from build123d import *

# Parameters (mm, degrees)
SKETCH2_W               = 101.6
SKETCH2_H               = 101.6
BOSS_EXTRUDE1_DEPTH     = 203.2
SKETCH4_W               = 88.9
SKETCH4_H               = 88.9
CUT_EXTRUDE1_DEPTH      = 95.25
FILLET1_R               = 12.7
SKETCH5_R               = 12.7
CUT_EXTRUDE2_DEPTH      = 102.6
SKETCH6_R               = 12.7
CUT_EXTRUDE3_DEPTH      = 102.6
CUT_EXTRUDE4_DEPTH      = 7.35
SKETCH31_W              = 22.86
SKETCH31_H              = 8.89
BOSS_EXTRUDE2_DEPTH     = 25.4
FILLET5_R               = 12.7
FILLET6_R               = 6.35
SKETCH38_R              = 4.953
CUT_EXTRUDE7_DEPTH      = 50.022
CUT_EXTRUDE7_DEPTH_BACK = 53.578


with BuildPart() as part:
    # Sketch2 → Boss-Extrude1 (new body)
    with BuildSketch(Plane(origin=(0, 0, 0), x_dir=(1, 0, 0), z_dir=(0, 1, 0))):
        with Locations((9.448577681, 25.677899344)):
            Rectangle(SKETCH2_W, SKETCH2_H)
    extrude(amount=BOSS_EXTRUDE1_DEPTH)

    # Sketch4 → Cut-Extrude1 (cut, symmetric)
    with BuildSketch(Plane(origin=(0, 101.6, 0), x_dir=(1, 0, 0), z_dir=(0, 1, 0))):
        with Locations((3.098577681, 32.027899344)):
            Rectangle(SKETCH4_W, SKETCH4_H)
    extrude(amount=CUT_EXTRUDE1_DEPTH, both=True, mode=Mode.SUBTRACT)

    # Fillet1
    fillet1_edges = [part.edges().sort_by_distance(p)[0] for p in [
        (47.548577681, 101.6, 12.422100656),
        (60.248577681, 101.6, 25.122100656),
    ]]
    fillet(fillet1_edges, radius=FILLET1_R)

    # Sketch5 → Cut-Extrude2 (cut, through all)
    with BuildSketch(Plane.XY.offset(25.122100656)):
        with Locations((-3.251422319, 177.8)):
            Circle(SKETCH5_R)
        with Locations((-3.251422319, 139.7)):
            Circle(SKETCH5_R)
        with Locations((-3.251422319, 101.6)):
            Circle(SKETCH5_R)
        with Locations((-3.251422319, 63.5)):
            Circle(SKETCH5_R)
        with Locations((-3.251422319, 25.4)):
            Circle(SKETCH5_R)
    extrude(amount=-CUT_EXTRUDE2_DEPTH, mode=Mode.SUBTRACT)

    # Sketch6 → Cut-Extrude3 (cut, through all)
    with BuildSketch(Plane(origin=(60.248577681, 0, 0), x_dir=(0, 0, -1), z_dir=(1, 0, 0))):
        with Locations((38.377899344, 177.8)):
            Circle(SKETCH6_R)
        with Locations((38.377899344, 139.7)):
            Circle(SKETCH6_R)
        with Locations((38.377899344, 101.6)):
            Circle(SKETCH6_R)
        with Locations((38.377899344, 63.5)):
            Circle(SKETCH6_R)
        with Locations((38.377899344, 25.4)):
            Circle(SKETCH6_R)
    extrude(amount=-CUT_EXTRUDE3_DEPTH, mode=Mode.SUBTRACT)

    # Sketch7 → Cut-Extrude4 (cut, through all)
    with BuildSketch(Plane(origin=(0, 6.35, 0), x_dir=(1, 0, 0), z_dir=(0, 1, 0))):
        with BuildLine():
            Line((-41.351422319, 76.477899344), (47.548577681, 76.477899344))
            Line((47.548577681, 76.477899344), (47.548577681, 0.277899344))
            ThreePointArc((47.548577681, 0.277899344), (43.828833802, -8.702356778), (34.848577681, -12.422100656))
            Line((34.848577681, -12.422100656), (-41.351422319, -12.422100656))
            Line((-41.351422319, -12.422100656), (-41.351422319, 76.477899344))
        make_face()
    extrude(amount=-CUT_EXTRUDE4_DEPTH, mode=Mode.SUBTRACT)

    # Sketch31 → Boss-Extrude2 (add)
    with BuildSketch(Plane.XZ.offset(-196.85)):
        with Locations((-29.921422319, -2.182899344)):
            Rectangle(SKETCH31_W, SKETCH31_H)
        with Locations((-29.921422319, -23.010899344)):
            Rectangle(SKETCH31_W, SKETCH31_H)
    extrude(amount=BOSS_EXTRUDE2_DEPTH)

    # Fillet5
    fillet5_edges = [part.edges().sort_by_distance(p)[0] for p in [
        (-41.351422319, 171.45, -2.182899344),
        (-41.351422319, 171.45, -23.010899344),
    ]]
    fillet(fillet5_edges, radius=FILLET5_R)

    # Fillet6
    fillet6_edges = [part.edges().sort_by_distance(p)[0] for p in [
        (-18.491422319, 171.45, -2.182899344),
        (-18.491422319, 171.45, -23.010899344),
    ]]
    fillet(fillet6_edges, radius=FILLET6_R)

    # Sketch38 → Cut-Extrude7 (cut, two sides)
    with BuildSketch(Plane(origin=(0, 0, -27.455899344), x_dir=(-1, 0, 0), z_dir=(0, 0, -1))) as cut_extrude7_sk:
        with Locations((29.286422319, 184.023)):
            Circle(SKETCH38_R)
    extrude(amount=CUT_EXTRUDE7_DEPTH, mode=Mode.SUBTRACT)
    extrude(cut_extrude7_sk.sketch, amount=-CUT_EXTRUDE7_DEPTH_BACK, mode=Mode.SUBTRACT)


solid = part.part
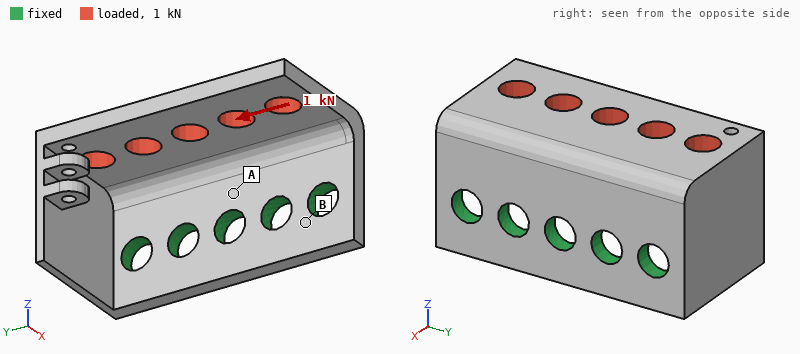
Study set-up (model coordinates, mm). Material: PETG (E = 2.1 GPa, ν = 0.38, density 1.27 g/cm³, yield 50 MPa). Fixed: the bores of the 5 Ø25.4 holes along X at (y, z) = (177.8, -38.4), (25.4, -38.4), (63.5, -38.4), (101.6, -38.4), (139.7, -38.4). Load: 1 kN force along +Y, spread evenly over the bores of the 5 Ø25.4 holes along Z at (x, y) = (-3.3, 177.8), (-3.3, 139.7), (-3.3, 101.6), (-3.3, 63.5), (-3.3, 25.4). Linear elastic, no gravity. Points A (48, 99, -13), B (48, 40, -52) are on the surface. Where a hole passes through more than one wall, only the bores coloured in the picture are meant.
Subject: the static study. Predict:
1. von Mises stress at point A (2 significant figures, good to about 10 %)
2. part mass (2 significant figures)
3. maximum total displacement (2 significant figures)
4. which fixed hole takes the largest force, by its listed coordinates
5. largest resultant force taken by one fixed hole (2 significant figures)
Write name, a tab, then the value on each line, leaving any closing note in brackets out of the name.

von Mises stress at point A	1.8 MPa
part mass	620 g
maximum total displacement	0.76 mm
which fixed hole takes the largest force, by its listed coordinates	(177.8, -38.4)
largest resultant force taken by one fixed hole	470 N
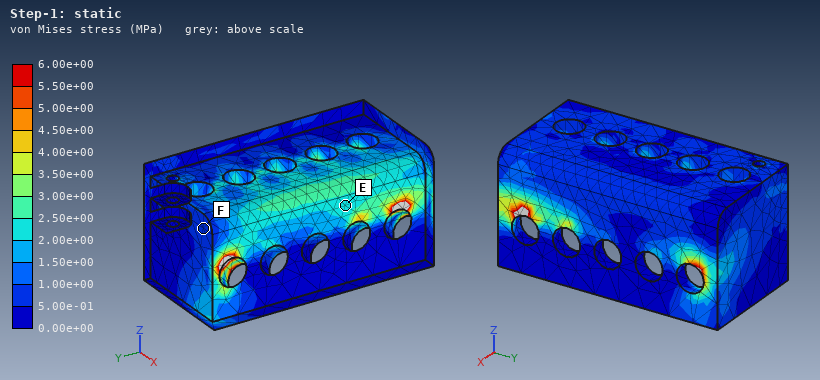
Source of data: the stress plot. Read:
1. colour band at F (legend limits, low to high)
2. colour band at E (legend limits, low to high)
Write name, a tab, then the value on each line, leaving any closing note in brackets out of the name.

colour band at F	5.00e-01 to 1.00e+00 MPa
colour band at E	2.00e+00 to 2.50e+00 MPa
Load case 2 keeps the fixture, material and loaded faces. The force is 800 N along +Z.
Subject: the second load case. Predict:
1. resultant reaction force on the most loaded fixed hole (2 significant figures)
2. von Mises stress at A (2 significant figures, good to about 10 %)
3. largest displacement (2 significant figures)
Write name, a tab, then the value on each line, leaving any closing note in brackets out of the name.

resultant reaction force on the most loaded fixed hole	210 N
von Mises stress at A	5.8 MPa
largest displacement	2.6 mm
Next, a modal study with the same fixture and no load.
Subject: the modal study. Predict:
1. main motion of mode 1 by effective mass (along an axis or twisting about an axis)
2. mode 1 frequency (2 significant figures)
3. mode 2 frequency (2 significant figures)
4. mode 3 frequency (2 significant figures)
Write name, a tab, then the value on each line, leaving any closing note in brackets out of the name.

main motion of mode 1 by effective mass	along Z
mode 1 frequency	220 Hz
mode 2 frequency	290 Hz
mode 3 frequency	350 Hz
